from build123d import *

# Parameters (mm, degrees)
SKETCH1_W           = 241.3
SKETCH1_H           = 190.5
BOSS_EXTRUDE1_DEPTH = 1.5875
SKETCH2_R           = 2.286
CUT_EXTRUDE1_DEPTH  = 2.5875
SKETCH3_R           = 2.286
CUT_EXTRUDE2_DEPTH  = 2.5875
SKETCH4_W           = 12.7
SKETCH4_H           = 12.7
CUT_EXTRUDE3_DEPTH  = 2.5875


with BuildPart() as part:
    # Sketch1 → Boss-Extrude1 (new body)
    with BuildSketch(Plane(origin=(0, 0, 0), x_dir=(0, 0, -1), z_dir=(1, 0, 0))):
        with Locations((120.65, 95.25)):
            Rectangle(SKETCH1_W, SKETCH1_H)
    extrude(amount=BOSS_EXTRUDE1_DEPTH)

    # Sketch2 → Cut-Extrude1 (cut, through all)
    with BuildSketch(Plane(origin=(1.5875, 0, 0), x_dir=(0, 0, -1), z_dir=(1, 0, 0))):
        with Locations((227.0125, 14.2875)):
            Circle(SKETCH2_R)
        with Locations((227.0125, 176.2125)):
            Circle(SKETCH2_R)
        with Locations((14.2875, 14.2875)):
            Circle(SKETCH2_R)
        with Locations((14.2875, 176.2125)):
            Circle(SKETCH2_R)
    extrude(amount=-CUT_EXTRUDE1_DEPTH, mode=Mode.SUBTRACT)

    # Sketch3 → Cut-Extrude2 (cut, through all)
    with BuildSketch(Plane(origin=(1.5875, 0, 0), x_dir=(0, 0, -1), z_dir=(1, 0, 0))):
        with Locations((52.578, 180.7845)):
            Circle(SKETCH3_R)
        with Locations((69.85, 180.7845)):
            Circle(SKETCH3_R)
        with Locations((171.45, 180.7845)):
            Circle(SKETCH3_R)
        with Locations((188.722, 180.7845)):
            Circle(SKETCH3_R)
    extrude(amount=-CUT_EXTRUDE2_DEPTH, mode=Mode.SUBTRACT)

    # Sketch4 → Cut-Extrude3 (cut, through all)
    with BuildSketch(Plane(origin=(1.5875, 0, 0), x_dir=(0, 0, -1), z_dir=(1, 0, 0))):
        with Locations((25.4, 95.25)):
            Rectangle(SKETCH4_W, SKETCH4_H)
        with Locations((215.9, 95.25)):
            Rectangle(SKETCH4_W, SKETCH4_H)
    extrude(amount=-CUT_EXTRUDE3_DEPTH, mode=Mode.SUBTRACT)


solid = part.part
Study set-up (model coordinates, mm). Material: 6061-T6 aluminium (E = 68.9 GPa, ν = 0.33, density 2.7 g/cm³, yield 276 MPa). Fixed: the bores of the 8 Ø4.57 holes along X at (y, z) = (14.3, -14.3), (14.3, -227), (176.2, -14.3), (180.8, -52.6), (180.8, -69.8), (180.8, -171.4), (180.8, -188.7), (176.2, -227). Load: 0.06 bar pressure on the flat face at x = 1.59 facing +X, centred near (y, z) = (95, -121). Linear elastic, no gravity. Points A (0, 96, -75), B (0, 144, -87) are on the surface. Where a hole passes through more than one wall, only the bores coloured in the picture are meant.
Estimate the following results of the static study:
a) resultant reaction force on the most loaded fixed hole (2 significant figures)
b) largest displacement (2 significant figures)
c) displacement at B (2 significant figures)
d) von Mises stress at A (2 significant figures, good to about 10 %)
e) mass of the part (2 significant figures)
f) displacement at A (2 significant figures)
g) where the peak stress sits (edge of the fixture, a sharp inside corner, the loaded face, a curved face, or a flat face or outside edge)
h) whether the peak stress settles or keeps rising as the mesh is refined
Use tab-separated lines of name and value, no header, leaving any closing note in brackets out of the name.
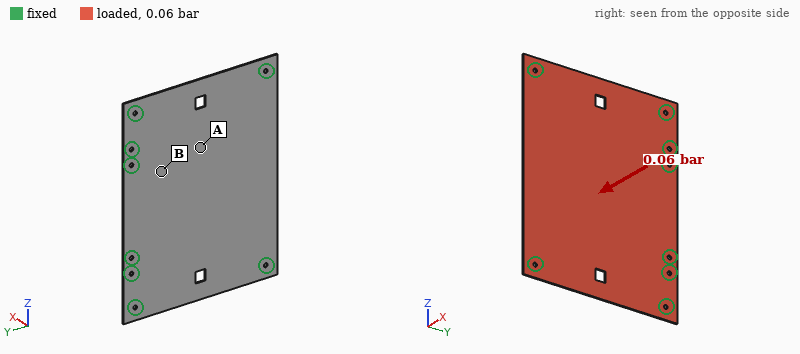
resultant reaction force on the most loaded fixed hole	63 N
largest displacement	1.8 mm
displacement at B	0.57 mm
von Mises stress at A	19 MPa
mass of the part	200 g
displacement at A	1.2 mm
where the peak stress sits	edge of the fixture
whether the peak stress settles or keeps rising as the mesh is refined	keeps rising
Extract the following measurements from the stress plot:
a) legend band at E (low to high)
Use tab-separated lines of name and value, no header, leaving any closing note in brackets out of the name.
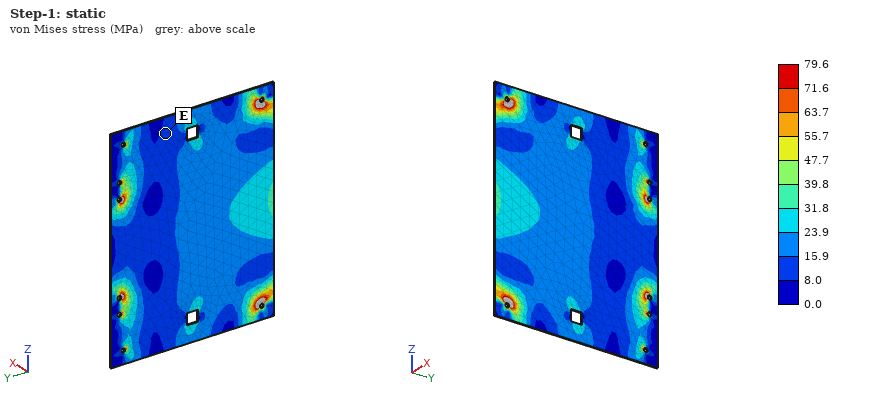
legend band at E	8.0 to 15.9 MPa
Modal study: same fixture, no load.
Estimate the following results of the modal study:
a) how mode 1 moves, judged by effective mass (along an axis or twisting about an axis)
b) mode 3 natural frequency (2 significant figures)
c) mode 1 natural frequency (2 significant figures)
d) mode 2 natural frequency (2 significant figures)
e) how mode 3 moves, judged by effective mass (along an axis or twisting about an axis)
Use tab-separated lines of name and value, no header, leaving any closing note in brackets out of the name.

how mode 1 moves, judged by effective mass	along X
mode 3 natural frequency	320 Hz
mode 1 natural frequency	170 Hz
mode 2 natural frequency	300 Hz
how mode 3 moves, judged by effective mass	twisting about Y
